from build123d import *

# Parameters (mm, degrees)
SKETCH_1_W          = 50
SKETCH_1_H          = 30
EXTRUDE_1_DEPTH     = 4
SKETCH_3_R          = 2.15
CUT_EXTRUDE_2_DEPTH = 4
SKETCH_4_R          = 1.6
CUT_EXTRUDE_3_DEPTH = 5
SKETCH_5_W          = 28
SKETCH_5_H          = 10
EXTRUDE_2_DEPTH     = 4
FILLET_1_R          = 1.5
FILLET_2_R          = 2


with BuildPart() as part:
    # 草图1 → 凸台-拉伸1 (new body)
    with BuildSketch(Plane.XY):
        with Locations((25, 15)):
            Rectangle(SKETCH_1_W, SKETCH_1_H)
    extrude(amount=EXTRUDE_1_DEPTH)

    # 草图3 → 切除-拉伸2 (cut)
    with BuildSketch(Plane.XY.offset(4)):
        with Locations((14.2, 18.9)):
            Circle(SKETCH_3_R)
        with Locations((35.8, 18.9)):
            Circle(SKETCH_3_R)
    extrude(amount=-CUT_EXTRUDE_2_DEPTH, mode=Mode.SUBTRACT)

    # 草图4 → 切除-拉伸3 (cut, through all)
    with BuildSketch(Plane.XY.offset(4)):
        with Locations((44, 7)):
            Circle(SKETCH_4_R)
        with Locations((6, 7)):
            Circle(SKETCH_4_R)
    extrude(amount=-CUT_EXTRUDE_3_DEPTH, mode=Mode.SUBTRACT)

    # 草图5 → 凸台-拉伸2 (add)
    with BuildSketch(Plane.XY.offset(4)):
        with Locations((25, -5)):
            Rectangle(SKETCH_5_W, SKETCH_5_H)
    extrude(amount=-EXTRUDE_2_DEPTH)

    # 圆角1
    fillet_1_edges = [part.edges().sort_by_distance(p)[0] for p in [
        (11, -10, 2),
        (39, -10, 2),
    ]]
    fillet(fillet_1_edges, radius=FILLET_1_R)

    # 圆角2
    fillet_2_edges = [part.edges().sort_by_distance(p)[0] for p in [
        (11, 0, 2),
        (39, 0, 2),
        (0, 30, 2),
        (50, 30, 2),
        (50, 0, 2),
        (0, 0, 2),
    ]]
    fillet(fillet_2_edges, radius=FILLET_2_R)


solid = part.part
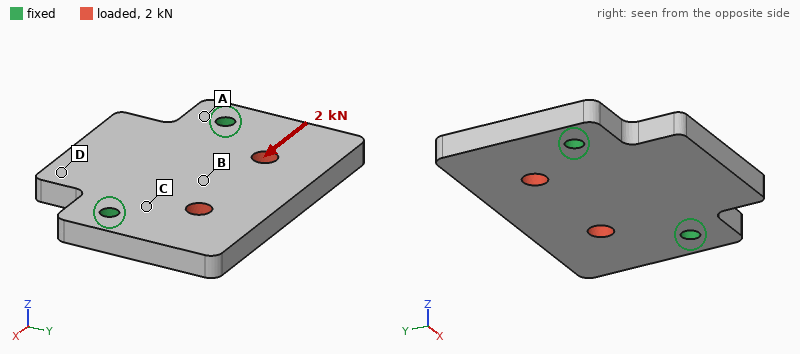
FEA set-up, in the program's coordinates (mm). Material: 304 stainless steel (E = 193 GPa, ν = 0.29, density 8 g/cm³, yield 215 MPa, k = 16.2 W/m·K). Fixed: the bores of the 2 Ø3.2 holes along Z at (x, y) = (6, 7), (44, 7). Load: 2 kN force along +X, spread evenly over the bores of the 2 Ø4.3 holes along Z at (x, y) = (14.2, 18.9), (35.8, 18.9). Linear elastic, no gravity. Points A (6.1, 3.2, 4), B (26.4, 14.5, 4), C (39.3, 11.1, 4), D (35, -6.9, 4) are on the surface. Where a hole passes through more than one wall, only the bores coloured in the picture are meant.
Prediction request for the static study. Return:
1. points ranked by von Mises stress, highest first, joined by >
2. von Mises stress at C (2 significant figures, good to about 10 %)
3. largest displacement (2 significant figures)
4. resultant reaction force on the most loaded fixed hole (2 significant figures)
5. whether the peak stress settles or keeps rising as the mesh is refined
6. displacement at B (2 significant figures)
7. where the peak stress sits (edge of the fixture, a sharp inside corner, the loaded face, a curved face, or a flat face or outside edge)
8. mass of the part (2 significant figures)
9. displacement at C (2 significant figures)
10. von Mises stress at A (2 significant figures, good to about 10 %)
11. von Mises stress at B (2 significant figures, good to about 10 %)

C > B > A > D
26 MPa
3.3 µm
1.2 kN
keeps rising
1.8 µm
edge of the fixture
55 g
0.97 µm
11 MPa
18 MPa
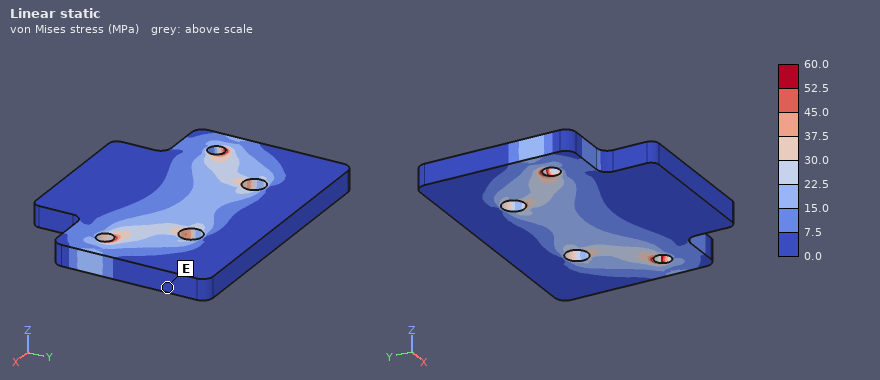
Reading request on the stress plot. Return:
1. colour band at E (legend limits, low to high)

0.0 to 7.5 MPa
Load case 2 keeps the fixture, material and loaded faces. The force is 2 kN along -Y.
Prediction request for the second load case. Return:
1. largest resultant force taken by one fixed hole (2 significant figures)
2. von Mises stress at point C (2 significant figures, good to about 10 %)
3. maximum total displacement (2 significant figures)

1.0 kN
21 MPa
2.3 µm
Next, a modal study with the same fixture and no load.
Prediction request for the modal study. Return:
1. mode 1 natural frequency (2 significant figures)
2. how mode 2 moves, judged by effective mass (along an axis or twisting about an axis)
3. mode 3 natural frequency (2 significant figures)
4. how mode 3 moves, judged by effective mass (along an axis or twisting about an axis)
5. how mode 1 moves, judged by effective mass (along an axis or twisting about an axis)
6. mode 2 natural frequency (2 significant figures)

4500 Hz
along Z
8400 Hz
twisting about Y
along Z
7700 Hz
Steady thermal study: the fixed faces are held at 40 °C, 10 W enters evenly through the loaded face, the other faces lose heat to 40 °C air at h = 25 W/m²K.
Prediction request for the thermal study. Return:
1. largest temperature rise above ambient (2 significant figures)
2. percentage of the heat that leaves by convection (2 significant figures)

57 K
28 %
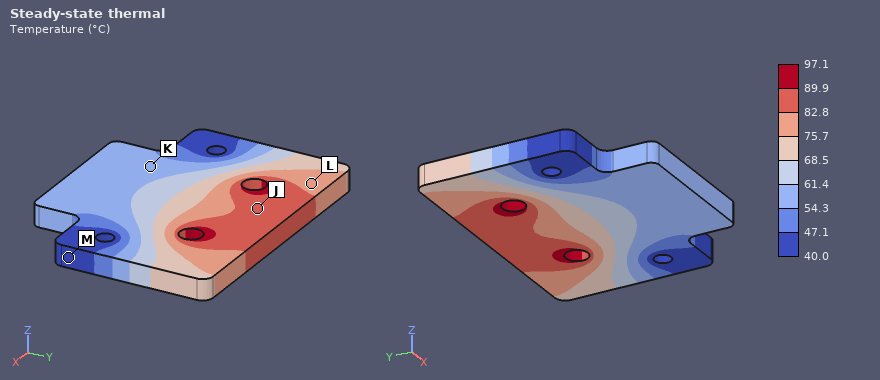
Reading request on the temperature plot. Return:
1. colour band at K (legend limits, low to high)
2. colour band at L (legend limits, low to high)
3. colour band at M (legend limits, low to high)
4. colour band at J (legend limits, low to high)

54.3 to 61.4 °C
75.7 to 82.8 °C
40.0 to 47.1 °C
82.8 to 89.9 °C
